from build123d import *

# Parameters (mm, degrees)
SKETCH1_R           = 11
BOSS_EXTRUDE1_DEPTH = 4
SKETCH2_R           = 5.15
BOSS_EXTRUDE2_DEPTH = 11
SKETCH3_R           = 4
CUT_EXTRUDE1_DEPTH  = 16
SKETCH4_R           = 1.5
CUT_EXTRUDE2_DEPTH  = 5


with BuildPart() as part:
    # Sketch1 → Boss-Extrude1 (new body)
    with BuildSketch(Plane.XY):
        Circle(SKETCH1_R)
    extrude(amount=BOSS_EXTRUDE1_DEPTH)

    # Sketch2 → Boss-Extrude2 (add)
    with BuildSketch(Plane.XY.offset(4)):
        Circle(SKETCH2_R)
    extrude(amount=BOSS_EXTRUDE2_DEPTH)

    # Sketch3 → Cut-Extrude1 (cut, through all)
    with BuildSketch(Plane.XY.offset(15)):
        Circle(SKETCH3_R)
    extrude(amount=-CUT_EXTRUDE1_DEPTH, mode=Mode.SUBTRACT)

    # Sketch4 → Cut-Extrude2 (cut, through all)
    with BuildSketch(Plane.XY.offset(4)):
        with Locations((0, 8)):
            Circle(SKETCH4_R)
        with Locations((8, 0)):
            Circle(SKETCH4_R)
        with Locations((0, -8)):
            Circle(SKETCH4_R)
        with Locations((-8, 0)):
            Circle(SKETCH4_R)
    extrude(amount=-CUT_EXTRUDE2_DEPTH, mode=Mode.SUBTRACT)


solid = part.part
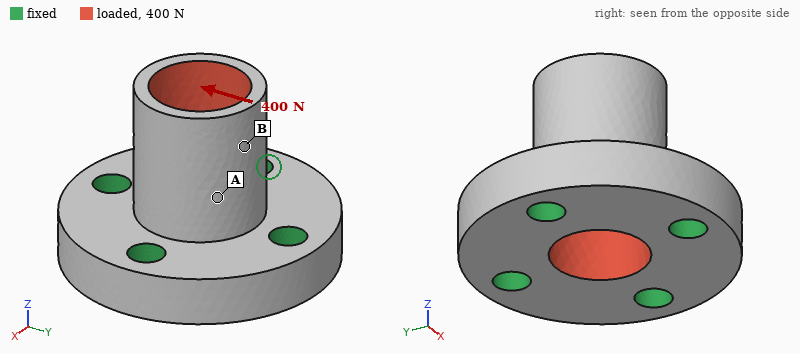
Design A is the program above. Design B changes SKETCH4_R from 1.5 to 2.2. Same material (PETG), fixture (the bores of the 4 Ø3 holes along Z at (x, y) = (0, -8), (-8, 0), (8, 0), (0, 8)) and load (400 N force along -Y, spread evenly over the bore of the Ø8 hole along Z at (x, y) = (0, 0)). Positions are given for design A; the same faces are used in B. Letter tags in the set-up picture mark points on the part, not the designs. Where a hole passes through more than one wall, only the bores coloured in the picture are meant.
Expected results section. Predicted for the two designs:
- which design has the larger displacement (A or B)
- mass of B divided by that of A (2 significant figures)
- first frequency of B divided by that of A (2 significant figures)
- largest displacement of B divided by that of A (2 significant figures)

A
0.92
1.0
0.92
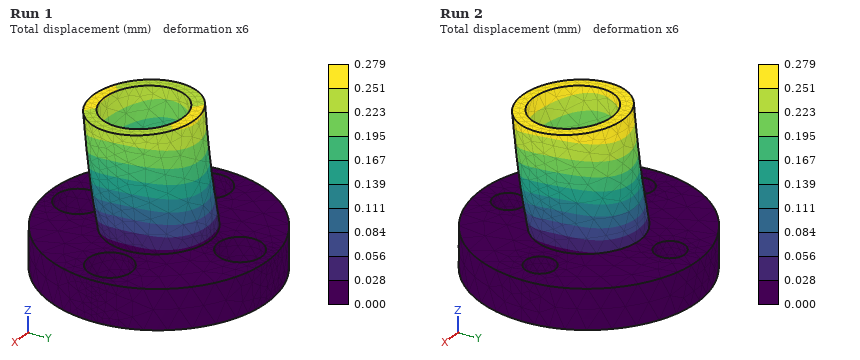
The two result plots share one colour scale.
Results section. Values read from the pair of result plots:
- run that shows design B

Run 1
